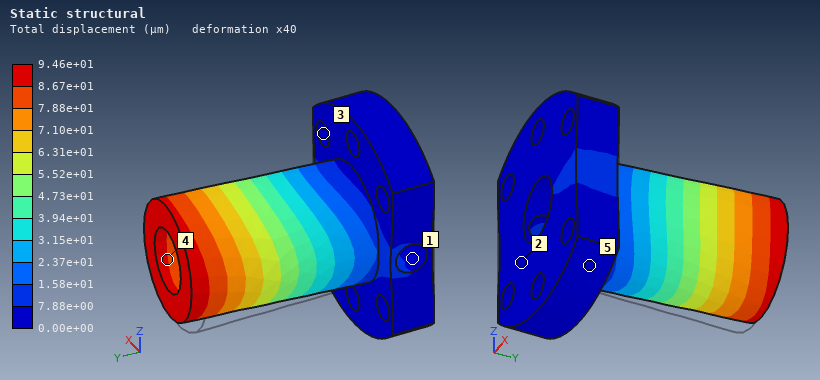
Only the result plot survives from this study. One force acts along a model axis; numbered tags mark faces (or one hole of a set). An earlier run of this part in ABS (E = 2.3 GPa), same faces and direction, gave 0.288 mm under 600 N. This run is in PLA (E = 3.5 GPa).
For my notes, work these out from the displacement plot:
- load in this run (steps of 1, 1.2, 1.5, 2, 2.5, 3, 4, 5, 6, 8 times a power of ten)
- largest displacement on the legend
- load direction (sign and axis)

300 N
9.46e+01 µm
+X
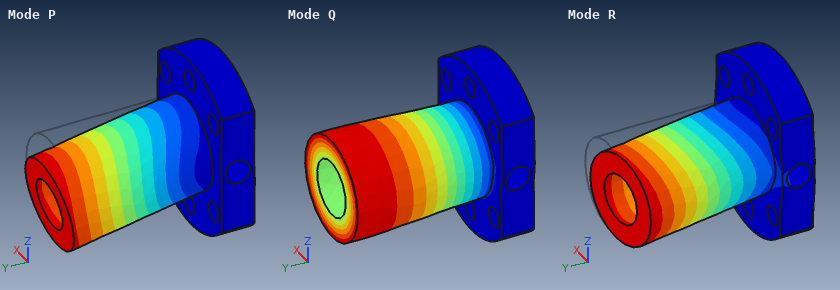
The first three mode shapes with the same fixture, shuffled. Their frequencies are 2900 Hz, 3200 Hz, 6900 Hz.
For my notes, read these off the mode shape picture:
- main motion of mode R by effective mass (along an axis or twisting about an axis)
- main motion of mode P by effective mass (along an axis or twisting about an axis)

along X
along Z
